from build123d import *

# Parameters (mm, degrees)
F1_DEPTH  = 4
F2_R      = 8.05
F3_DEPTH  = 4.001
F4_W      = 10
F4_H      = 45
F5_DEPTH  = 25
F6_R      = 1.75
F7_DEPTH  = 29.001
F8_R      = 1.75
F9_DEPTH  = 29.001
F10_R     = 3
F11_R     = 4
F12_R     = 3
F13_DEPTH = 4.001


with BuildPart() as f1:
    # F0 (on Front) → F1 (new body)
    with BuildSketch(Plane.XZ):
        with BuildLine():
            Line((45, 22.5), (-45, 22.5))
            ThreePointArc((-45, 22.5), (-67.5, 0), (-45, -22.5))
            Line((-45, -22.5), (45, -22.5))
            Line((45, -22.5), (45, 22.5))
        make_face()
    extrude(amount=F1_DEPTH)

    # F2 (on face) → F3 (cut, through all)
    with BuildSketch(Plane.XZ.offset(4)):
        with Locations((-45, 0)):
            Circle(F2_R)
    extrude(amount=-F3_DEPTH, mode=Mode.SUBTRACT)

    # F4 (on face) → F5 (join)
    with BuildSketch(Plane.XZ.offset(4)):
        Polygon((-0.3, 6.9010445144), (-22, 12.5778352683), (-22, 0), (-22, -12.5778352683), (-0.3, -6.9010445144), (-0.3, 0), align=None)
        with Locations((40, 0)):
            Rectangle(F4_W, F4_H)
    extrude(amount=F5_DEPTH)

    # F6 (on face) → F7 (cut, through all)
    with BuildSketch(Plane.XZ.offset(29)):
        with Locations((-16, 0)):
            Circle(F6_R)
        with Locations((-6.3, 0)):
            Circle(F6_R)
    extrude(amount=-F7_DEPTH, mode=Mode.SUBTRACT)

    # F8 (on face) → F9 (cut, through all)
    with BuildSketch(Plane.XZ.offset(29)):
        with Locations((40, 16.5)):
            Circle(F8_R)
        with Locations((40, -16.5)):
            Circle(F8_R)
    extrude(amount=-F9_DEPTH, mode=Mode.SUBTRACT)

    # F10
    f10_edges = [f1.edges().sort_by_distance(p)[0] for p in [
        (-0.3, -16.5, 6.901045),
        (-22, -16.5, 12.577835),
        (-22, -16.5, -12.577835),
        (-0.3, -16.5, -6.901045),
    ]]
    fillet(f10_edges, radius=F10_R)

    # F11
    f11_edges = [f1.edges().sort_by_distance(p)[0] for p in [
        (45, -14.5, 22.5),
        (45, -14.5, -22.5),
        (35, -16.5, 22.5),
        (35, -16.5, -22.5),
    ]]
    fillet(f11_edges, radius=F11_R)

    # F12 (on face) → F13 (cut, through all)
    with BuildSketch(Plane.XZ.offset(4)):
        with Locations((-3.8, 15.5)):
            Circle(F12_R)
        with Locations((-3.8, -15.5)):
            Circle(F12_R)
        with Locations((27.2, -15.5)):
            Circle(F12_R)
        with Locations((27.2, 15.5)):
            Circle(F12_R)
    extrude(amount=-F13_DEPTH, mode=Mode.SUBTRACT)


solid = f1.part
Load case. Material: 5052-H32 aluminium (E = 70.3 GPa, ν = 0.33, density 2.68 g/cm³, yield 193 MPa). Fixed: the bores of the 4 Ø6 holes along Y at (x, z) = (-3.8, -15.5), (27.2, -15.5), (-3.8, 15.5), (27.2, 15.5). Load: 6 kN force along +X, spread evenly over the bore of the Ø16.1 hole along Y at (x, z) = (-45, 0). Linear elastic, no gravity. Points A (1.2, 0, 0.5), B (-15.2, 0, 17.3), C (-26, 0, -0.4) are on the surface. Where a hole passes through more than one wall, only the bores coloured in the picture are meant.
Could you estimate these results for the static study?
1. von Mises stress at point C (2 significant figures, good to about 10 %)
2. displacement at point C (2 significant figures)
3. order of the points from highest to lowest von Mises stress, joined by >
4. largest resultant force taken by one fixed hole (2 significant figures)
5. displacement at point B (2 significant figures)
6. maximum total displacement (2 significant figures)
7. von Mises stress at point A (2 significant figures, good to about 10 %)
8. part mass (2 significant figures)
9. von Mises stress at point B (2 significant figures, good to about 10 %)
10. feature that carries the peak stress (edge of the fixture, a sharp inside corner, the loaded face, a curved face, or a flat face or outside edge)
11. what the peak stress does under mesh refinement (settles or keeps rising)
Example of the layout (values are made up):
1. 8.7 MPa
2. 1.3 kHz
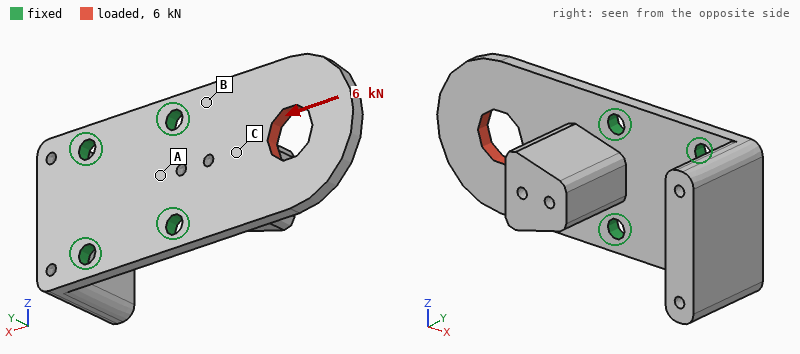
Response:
1. 30 MPa
2. 14 µm
3. B > C > A
4. 2.7 kN
5. 6.6 µm
6. 43 µm
7. 11 MPa
8. 100 g
9. 44 MPa
10. a sharp inside corner
11. keeps rising
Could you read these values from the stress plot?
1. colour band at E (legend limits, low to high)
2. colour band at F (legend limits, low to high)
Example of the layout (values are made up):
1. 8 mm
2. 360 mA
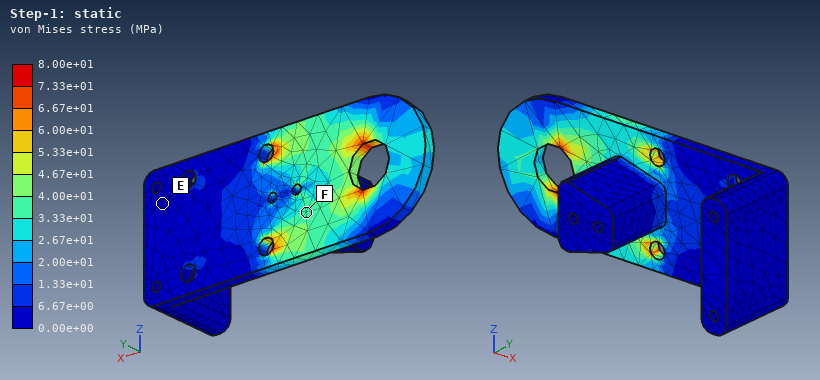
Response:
1. 0.00e+00 to 6.67e+00 MPa
2. 3.33e+01 to 4.00e+01 MPa
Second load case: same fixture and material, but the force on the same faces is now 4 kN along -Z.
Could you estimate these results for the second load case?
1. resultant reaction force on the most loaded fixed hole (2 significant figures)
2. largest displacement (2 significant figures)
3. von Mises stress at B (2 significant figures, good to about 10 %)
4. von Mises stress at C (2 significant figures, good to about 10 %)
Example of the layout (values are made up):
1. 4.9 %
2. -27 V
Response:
1. 5.0 kN
2. 0.13 mm
3. 72 MPa
4. 76 MPa
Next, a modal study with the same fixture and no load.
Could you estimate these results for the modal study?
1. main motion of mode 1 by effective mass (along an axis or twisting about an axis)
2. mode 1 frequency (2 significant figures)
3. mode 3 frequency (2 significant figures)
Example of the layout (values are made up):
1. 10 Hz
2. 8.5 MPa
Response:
1. along Y
2. 1300 Hz
3. 3700 Hz
